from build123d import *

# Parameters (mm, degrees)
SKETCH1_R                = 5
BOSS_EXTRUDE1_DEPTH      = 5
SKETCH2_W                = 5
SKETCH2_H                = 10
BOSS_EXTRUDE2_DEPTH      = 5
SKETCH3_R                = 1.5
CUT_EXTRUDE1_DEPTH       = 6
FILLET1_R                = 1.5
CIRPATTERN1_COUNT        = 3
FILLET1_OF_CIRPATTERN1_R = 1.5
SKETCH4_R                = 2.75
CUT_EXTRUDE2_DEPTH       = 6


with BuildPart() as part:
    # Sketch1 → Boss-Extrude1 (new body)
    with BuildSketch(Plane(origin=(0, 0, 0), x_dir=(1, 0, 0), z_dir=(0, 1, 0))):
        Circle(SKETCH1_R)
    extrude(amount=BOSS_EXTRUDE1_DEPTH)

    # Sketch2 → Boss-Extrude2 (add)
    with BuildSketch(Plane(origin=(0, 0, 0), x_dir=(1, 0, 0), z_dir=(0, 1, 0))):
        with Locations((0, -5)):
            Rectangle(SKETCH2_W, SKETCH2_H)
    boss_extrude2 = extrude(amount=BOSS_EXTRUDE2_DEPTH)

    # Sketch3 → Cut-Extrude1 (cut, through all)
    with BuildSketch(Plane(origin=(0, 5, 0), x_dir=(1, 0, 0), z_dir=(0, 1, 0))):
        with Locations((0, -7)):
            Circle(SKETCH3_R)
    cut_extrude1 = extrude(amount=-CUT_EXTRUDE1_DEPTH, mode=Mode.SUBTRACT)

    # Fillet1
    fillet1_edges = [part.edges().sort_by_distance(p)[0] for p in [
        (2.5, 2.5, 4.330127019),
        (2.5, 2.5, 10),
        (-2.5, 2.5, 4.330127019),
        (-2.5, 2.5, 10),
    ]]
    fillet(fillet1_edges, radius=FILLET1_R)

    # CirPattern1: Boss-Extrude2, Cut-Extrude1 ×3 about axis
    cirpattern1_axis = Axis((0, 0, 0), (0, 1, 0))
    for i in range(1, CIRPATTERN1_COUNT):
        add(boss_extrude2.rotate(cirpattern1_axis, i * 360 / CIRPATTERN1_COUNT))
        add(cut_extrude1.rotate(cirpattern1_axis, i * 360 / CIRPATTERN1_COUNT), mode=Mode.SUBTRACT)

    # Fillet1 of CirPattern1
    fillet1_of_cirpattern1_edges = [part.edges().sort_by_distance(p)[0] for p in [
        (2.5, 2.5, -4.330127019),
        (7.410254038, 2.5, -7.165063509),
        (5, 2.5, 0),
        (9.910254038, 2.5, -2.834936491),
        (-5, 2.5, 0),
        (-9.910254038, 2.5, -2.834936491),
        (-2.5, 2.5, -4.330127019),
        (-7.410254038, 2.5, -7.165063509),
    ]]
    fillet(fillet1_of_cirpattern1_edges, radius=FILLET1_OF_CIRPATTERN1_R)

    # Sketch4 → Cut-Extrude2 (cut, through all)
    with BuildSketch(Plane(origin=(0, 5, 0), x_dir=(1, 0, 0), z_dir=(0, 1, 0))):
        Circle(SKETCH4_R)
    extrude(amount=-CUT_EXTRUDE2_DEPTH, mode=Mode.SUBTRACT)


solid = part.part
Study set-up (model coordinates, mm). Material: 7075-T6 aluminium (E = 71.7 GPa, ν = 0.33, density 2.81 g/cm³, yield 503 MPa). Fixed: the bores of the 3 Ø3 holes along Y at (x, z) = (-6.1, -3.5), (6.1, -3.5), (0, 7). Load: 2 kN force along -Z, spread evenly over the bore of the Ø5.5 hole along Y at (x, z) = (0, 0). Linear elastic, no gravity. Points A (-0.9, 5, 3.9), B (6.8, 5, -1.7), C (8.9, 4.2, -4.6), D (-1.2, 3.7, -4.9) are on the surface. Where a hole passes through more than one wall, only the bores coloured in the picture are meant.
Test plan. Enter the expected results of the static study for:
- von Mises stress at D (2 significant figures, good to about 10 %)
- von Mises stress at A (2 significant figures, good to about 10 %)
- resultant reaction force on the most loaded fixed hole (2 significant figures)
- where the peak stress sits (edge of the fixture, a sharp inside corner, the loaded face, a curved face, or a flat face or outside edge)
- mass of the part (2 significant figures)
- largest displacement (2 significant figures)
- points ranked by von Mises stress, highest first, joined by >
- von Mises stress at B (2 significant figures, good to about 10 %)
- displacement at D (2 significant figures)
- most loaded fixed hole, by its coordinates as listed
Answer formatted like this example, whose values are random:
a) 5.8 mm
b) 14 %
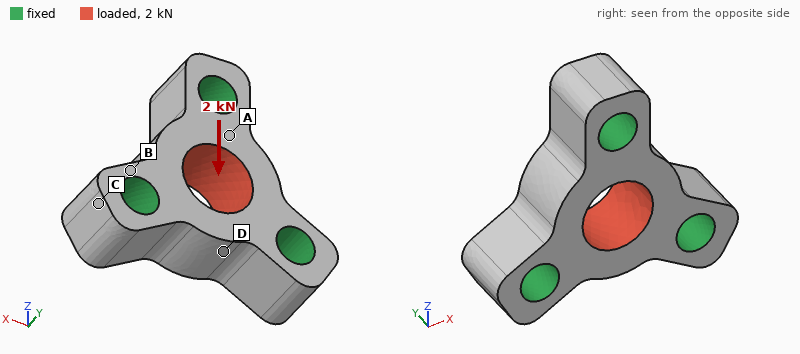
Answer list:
a) 44 MPa
b) 30 MPa
c) 730 N
d) edge of the fixture
e) 1.5 g
f) 6.5 µm
g) D > A > B > C
h) 17 MPa
i) 5.1 µm
j) (0, 7)
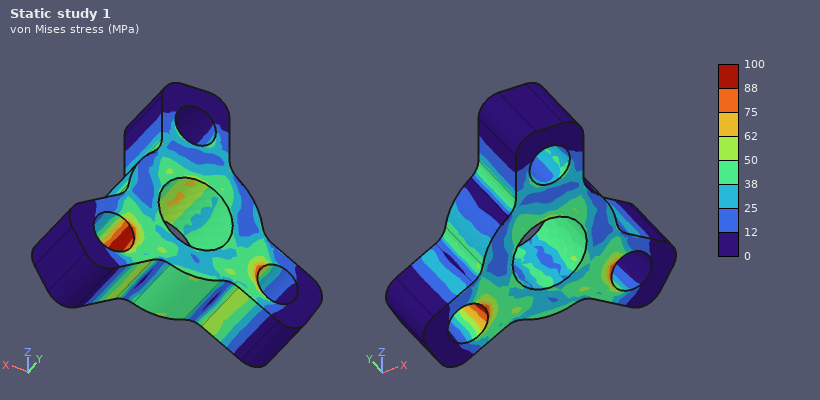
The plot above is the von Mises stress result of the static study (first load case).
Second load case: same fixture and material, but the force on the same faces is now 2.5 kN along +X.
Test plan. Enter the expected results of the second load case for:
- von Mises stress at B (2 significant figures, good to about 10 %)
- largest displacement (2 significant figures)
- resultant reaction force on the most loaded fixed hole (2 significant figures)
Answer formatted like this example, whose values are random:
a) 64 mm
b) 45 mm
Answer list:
a) 40 MPa
b) 7.1 µm
c) 880 N
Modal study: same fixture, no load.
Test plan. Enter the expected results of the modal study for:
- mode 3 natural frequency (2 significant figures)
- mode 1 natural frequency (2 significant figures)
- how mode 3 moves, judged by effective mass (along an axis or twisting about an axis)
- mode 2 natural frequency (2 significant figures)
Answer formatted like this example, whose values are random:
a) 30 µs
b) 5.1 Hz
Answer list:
a) 140 kHz
b) 130 kHz
c) along Y
d) 130 kHz
